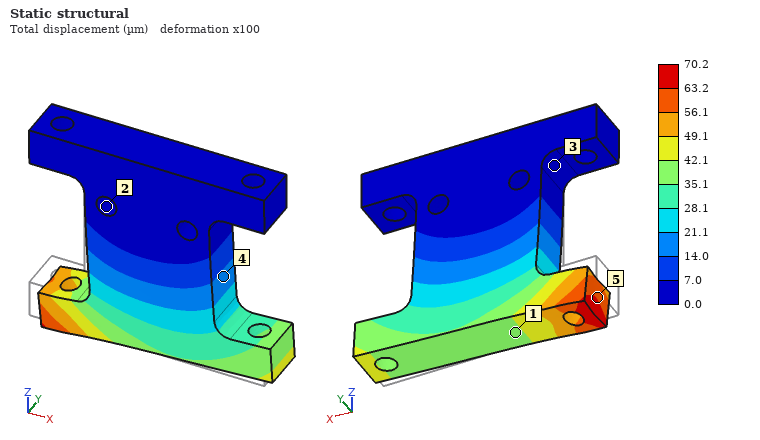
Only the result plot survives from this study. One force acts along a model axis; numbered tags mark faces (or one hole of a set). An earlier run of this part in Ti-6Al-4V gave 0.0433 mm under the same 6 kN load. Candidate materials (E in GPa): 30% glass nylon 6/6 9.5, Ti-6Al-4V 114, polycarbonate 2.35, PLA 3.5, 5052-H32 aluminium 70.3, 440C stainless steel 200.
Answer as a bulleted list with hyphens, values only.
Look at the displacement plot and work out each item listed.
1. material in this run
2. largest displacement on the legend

- 5052-H32 aluminium
- 70.2 µm
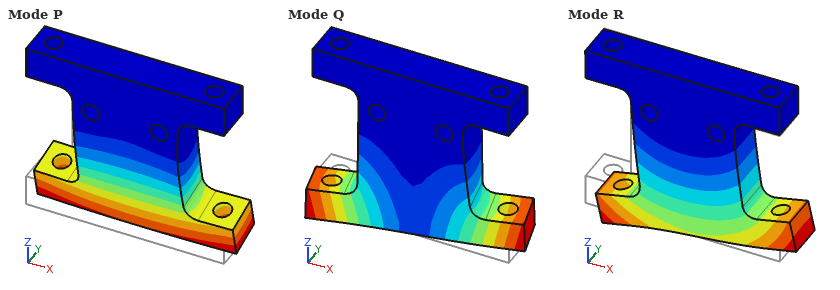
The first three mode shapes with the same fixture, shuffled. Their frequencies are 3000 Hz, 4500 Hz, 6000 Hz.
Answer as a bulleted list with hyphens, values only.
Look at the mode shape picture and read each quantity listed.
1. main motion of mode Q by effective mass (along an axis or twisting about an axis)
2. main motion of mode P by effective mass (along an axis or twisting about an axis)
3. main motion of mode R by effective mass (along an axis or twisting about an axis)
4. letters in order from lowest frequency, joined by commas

- twisting about Z
- along Y
- along X
- P, Q, R
